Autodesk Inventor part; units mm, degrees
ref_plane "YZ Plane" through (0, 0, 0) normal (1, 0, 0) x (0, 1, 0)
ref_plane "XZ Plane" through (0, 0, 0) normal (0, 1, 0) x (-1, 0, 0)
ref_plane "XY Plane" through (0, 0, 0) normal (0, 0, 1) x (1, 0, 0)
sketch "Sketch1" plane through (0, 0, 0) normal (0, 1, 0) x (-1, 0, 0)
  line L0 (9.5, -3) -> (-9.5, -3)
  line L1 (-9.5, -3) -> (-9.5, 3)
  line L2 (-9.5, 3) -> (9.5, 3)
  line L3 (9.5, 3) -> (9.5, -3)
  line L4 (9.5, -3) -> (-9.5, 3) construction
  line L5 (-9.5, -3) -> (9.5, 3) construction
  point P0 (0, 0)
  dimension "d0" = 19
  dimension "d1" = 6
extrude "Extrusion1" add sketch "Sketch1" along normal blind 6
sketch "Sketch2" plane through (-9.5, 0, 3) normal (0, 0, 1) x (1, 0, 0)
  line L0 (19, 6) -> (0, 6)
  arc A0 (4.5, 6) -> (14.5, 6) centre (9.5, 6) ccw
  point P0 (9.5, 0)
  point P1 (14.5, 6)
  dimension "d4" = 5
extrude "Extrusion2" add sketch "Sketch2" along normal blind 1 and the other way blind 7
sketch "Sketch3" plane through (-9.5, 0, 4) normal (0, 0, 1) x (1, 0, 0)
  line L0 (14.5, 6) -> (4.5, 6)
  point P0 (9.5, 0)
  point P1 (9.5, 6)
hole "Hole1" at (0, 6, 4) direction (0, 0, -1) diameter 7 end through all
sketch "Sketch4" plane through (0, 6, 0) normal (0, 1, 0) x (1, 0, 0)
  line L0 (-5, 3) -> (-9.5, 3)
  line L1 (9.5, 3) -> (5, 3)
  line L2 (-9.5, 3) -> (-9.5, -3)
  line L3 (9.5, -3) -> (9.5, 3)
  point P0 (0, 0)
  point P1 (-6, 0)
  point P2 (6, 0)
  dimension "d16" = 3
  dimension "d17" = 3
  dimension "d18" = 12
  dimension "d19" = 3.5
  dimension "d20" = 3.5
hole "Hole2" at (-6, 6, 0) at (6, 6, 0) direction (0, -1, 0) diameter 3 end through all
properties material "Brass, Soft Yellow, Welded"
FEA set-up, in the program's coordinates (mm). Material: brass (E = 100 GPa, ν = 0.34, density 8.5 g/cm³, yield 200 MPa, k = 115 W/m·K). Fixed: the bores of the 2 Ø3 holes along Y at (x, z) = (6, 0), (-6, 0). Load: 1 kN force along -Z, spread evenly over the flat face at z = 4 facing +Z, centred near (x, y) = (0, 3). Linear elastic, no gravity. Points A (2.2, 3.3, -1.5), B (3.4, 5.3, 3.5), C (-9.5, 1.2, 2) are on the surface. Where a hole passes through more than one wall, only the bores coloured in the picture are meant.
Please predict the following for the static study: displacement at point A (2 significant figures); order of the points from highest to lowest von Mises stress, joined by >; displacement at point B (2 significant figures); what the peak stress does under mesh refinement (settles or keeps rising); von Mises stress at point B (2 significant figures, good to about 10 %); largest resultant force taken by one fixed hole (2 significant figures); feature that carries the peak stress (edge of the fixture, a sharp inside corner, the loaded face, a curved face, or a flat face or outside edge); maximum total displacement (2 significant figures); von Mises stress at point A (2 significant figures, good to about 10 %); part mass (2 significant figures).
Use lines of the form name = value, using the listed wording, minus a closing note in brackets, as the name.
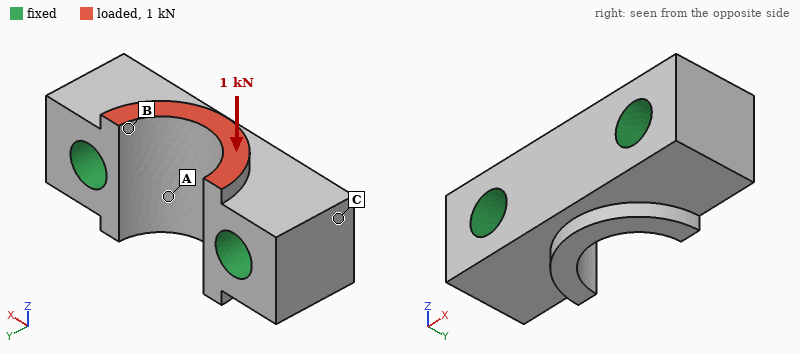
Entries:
displacement at point A = 0.88 µm
order of the points from highest to lowest von Mises stress, joined by > = B > A > C
displacement at point B = 2.4 µm
what the peak stress does under mesh refinement = keeps rising
von Mises stress at point B = 52 MPa
largest resultant force taken by one fixed hole = 510 N
feature that carries the peak stress = edge of the fixture
maximum total displacement = 2.9 µm
von Mises stress at point A = 14 MPa
part mass = 4.5 g
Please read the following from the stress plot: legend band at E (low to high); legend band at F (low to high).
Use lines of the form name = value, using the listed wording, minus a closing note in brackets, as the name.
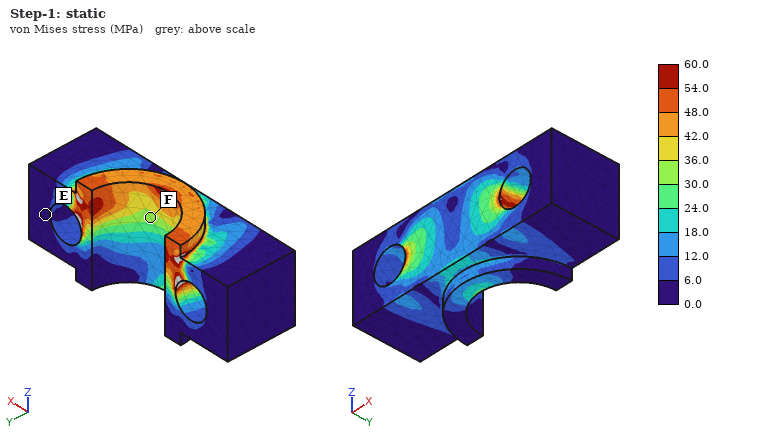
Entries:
legend band at E = 0.0 to 6.0 MPa
legend band at F = 30.0 to 36.0 MPa
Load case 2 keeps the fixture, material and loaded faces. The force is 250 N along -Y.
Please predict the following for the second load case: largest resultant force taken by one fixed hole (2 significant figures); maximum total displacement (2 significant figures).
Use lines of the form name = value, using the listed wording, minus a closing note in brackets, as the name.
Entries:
largest resultant force taken by one fixed hole = 130 N
maximum total displacement = 2.8 µm
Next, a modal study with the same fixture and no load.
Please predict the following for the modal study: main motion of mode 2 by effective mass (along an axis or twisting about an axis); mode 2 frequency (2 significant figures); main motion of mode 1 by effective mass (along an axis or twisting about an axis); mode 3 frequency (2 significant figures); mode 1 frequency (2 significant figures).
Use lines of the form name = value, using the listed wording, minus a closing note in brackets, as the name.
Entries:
main motion of mode 2 by effective mass = along Y
mode 2 frequency = 93 kHz
main motion of mode 1 by effective mass = along Z
mode 3 frequency = 110 kHz
mode 1 frequency = 85 kHz
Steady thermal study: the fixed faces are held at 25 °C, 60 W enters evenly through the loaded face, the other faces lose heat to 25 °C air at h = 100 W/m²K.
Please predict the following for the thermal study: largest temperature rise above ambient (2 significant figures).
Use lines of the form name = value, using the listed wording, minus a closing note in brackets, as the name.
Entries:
largest temperature rise above ambient = 77 K
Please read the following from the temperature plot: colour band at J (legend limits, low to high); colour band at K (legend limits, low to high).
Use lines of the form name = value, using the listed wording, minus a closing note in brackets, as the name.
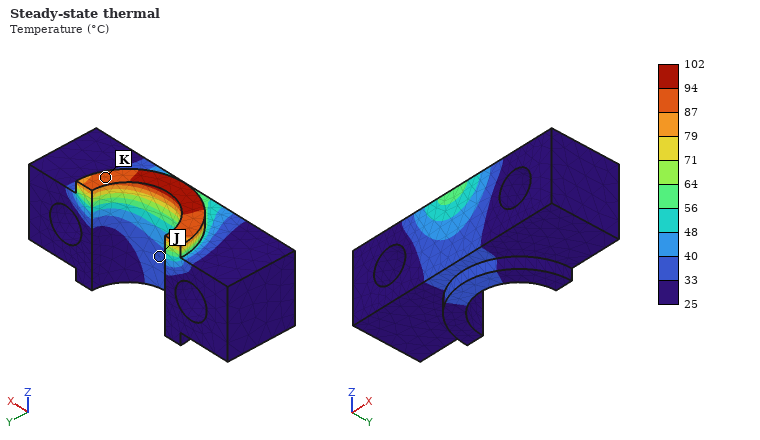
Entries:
colour band at J = 33 to 40 °C
colour band at K = 87 to 94 °C
